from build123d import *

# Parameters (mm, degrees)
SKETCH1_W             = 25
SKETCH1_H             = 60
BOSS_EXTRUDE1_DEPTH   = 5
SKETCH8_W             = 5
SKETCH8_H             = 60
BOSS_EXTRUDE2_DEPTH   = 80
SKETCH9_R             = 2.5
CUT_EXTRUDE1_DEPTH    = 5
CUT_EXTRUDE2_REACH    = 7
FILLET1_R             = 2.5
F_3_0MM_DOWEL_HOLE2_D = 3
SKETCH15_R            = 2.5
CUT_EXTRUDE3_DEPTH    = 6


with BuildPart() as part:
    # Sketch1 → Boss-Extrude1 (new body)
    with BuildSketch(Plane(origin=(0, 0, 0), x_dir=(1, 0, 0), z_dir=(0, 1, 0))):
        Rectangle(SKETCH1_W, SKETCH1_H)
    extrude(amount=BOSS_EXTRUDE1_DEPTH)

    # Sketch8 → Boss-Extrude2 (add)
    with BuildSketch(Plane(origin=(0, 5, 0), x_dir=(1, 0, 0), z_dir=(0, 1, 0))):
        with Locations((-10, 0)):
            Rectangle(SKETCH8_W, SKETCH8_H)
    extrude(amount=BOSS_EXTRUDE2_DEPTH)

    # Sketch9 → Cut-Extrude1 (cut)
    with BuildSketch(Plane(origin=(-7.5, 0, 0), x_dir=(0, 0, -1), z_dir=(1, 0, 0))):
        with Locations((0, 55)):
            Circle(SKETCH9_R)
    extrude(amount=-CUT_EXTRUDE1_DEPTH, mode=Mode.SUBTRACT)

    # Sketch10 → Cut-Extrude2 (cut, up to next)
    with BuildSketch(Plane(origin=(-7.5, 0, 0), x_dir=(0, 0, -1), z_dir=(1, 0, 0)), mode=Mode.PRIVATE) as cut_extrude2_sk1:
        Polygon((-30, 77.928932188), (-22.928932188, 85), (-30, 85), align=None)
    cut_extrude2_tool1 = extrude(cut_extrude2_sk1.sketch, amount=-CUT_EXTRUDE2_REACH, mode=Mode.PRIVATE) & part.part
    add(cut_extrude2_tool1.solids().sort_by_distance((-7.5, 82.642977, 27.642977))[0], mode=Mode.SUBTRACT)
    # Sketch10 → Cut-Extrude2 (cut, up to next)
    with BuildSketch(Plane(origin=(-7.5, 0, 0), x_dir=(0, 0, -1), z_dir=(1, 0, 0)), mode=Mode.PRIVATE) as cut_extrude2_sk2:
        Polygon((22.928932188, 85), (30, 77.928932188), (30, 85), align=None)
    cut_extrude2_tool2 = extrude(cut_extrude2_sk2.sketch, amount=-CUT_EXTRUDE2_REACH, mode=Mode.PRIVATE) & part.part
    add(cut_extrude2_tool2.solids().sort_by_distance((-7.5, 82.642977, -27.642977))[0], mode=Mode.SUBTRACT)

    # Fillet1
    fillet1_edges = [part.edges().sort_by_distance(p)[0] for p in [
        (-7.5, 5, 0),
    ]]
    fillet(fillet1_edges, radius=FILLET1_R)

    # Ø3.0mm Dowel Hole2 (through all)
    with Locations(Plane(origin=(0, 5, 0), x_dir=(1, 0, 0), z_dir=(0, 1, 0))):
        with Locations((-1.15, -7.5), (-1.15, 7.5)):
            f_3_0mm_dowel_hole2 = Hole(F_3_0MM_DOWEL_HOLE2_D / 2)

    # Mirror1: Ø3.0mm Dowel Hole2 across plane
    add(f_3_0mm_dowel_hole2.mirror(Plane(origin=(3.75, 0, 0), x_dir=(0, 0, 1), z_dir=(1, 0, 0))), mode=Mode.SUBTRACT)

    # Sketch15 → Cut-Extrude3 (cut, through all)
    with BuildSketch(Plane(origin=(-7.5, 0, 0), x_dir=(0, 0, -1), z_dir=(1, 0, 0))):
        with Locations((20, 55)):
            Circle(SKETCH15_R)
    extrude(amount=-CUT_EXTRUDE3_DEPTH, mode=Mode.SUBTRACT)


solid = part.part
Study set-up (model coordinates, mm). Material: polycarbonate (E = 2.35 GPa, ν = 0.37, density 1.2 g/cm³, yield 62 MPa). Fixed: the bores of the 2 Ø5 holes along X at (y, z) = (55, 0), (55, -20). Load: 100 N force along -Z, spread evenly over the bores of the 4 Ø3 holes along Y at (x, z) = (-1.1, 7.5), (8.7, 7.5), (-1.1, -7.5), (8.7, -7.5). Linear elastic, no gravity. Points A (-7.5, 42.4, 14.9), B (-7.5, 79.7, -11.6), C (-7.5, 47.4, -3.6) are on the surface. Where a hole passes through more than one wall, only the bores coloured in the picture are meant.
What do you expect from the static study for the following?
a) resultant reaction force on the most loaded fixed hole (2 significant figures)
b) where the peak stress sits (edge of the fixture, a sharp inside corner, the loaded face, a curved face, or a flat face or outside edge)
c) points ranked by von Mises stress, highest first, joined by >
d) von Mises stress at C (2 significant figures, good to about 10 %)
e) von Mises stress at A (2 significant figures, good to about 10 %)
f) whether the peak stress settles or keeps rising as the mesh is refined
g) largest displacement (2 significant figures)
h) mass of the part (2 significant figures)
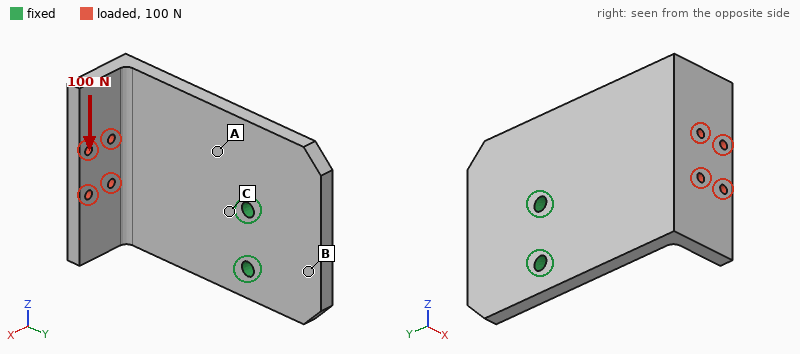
240 N
edge of the fixture
C > A > B
5.3 MPa
2.7 MPa
keeps rising
1.1 mm
37 g
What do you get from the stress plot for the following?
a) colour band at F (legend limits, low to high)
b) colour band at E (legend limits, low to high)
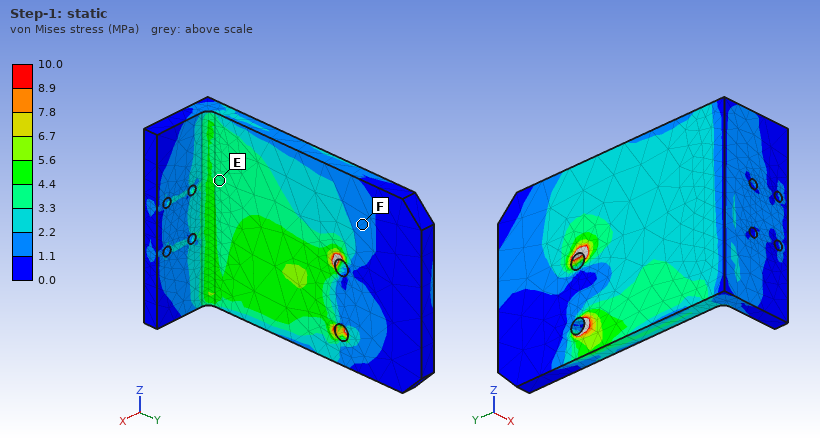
1.1 to 2.2 MPa
3.3 to 4.4 MPa
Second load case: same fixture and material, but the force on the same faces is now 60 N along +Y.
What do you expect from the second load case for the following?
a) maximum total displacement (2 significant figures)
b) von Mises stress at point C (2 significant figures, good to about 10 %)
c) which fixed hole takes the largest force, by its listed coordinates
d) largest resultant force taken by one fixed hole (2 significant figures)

1.1 mm
4.0 MPa
(55, 0)
56 N
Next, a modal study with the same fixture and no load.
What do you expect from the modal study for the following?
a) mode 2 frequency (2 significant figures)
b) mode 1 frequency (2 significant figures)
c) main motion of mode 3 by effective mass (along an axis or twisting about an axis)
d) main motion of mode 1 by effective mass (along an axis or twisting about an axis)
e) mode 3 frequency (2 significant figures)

480 Hz
230 Hz
along X
along X
1000 Hz
